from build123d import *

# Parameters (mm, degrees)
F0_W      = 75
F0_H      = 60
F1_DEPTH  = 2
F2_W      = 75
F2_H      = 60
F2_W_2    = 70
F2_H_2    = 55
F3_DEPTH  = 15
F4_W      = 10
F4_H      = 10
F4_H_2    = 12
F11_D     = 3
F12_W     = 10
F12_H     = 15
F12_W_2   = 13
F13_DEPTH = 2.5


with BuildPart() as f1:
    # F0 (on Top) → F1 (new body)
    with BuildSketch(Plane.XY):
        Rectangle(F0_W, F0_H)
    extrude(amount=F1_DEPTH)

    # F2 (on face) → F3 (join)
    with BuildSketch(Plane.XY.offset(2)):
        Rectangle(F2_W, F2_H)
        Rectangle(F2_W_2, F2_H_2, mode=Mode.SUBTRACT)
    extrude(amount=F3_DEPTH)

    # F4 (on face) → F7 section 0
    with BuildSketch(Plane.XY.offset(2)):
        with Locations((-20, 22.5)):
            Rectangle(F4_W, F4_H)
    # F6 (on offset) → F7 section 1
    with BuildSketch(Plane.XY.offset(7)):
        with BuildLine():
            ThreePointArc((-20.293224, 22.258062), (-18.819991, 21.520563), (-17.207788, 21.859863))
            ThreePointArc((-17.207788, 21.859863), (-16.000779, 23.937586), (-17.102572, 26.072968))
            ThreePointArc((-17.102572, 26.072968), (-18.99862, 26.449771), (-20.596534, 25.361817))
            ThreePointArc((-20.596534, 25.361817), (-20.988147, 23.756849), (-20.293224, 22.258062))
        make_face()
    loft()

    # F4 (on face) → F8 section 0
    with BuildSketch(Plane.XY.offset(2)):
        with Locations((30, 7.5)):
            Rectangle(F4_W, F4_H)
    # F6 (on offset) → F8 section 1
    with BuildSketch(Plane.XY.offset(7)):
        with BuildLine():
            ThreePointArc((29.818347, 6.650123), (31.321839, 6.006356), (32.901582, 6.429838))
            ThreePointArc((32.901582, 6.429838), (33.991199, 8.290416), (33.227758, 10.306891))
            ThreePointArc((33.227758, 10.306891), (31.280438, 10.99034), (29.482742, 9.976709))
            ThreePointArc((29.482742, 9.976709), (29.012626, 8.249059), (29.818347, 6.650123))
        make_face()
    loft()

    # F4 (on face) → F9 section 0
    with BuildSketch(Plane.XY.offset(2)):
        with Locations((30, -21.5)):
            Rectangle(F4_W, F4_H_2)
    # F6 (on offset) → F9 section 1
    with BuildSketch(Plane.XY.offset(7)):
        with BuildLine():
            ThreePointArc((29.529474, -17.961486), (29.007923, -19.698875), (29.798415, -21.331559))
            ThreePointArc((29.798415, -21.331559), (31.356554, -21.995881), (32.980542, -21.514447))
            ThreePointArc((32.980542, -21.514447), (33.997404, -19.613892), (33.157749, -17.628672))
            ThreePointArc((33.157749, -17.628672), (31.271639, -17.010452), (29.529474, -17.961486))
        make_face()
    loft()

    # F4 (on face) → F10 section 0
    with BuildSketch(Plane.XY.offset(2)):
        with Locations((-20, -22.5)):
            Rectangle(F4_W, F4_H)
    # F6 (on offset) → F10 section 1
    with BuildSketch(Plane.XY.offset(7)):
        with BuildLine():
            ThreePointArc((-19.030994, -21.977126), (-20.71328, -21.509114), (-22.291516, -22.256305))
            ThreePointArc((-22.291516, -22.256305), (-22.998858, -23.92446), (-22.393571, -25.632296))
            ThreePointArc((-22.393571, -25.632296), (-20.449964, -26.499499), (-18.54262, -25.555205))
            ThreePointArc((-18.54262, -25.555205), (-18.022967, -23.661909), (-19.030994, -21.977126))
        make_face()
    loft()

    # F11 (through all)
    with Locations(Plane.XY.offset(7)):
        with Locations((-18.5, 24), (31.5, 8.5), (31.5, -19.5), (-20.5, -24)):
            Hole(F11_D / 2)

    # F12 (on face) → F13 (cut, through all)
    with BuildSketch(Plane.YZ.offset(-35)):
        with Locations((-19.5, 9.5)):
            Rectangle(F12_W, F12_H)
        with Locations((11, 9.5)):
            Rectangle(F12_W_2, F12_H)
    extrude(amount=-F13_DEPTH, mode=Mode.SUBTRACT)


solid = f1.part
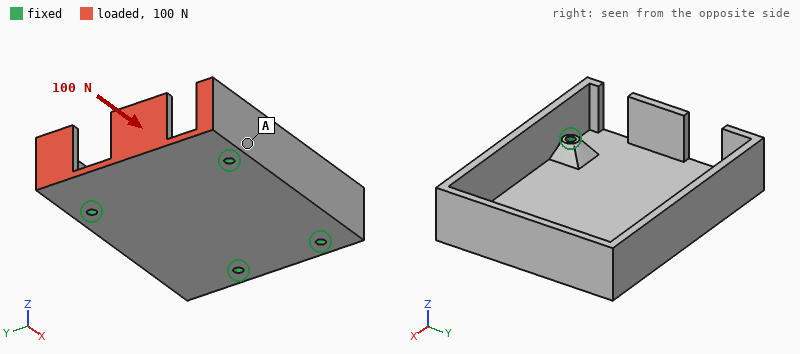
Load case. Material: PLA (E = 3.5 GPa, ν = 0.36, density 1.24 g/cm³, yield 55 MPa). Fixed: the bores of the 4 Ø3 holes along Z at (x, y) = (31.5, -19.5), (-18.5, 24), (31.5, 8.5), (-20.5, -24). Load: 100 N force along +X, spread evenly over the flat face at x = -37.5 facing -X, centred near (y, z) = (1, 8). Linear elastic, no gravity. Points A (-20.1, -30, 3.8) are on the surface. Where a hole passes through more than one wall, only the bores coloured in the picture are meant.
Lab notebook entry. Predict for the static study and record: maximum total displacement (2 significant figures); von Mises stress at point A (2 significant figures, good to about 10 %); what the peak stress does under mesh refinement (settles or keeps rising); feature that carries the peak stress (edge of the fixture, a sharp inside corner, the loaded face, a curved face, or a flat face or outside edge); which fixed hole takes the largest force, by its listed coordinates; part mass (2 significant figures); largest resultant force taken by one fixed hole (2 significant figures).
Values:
0.98 mm
1.8 MPa
keeps rising
a sharp inside corner
(-18.5, 24)
23 g
40 N
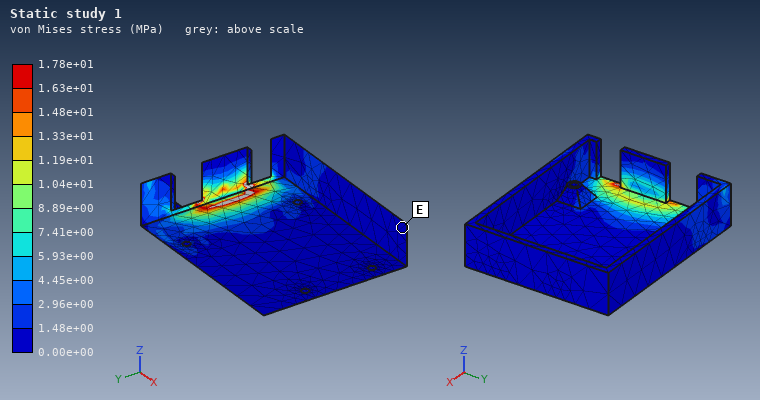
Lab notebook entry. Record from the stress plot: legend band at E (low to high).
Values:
0.00e+00 to 1.48e+00 MPa
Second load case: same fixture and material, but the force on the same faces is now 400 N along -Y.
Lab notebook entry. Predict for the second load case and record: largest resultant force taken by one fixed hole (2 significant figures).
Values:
260 N
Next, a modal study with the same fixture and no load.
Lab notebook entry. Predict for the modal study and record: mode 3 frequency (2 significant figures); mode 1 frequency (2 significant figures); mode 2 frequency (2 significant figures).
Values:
1700 Hz
1100 Hz
1600 Hz
